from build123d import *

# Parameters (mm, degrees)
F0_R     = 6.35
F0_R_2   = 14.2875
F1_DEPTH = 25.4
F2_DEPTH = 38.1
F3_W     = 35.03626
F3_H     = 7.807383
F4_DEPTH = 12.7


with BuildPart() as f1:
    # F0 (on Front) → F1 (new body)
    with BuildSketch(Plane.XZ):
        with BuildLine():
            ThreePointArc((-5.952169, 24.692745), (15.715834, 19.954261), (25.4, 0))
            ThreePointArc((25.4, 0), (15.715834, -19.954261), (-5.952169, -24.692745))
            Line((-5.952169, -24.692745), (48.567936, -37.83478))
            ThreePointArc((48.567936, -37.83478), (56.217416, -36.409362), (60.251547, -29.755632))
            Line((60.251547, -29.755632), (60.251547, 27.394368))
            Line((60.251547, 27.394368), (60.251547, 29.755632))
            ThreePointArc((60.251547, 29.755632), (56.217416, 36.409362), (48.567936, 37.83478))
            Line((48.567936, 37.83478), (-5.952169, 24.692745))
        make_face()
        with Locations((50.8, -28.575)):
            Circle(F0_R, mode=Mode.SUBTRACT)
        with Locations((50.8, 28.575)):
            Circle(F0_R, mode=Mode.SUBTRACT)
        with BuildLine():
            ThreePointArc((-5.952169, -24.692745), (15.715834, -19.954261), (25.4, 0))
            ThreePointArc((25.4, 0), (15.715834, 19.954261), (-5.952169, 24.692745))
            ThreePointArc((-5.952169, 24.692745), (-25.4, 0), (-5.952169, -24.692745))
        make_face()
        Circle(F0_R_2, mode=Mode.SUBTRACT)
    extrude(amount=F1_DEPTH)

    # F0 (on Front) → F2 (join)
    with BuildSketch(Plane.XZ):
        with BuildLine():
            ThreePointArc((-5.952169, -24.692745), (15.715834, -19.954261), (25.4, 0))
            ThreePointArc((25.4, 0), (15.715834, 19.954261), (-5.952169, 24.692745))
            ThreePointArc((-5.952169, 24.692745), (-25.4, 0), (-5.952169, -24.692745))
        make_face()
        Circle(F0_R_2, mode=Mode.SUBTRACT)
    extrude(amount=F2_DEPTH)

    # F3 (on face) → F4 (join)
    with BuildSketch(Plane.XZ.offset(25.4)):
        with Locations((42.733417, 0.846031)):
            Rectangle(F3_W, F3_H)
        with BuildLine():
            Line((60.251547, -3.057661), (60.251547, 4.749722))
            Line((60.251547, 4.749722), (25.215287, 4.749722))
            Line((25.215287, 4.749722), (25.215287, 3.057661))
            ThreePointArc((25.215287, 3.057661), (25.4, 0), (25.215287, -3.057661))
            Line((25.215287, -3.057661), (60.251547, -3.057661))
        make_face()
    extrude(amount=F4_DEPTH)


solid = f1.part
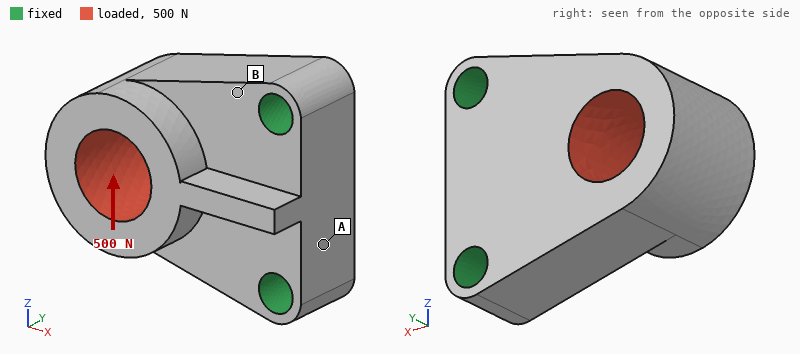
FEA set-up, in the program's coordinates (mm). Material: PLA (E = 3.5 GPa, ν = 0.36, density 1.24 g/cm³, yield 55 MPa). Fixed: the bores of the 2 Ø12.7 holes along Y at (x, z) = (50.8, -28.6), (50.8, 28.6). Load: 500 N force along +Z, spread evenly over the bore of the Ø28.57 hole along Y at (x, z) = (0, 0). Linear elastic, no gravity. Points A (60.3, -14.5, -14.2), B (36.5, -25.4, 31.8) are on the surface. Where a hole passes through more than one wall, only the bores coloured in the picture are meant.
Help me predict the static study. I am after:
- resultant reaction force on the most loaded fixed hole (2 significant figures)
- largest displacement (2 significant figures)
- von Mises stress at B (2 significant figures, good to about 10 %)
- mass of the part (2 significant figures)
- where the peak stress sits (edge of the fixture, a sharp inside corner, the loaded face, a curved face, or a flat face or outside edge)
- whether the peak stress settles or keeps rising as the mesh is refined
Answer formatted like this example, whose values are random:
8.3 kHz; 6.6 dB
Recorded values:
480 N; 41 µm; 0.79 MPa; 150 g; edge of the fixture; keeps rising
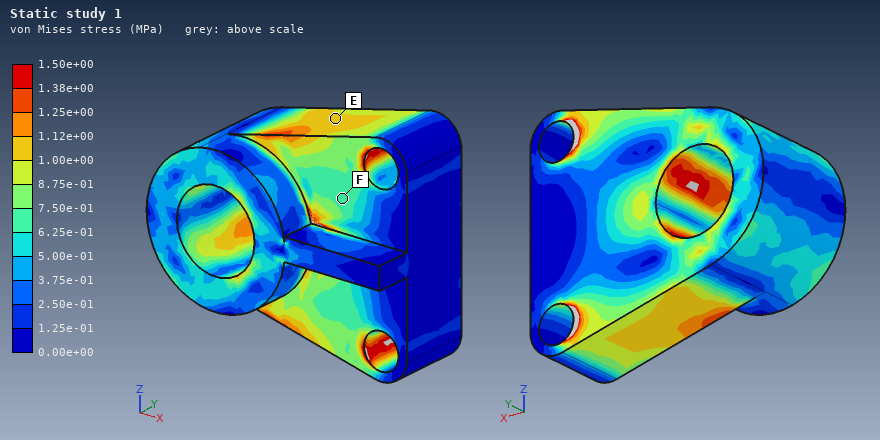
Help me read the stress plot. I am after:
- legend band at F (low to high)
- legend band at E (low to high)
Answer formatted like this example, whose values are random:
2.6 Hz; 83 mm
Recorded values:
6.25e-01 to 7.50e-01 MPa; 1.00e+00 to 1.12e+00 MPa
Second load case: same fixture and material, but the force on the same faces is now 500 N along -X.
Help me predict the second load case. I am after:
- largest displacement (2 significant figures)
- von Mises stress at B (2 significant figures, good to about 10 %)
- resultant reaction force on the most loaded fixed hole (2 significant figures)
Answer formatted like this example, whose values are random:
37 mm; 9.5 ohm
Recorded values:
32 µm; 0.80 MPa; 260 N
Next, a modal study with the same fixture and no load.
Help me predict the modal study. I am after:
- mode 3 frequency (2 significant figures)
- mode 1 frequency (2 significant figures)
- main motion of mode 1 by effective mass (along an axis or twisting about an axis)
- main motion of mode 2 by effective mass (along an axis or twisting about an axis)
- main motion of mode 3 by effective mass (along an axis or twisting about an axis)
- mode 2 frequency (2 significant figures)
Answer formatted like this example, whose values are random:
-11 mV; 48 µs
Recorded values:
3000 Hz; 1300 Hz; along Y; along Z; twisting about X; 2400 Hz
